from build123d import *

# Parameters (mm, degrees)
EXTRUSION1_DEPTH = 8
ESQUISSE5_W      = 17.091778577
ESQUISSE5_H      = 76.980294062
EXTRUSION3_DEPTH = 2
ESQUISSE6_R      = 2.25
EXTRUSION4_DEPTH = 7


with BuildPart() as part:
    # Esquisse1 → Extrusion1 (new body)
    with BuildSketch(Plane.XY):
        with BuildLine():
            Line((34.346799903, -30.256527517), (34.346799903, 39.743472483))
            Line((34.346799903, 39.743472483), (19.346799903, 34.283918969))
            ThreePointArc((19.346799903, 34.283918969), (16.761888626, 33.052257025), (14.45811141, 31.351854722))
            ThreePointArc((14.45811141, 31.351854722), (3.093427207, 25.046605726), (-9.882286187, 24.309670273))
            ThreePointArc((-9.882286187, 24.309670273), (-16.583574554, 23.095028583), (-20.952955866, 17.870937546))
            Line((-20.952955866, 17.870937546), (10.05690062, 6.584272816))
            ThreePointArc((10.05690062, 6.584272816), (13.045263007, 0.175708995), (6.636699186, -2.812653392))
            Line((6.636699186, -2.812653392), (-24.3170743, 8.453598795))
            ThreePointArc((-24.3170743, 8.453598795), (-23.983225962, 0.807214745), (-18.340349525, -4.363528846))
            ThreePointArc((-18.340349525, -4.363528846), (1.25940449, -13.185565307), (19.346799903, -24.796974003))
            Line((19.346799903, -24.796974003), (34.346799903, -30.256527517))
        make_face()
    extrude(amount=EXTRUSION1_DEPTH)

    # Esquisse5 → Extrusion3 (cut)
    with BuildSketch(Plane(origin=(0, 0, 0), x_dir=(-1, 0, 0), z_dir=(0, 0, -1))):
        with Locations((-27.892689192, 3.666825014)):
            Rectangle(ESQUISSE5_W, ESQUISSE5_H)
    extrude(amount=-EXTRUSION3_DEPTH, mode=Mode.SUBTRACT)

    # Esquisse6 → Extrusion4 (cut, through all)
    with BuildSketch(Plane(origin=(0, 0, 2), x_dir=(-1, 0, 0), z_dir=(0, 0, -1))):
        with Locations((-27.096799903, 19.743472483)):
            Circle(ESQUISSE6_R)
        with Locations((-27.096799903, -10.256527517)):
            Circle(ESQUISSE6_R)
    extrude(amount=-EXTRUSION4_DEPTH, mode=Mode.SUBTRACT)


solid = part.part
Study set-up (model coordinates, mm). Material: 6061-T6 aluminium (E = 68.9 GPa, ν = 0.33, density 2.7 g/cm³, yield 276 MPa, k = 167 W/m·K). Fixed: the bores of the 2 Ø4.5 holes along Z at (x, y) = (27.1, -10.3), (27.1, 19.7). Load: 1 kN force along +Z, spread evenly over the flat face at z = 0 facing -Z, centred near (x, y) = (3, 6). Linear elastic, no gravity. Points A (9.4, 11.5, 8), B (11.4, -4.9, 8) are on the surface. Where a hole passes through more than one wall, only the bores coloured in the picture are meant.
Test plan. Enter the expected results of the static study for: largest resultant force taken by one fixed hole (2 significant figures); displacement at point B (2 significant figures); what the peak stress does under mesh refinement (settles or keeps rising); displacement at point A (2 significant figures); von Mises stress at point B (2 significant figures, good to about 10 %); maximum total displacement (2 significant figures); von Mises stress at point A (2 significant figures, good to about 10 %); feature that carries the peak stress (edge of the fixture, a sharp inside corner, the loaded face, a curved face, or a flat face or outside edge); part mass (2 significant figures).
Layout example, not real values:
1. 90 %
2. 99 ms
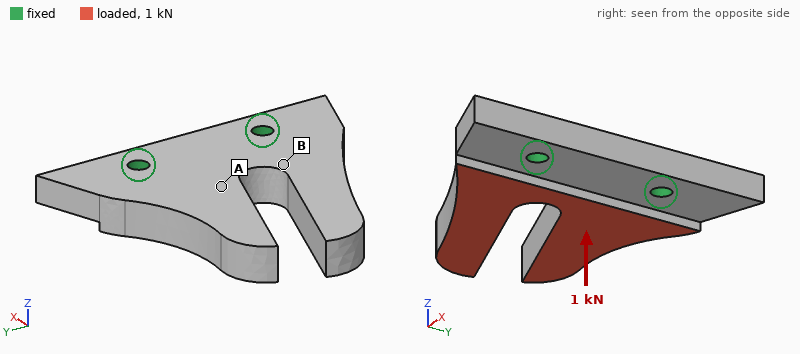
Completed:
1. 520 N
2. 0.049 mm
3. keeps rising
4. 0.050 mm
5. 43 MPa
6. 0.27 mm
7. 14 MPa
8. edge of the fixture
9. 42 g
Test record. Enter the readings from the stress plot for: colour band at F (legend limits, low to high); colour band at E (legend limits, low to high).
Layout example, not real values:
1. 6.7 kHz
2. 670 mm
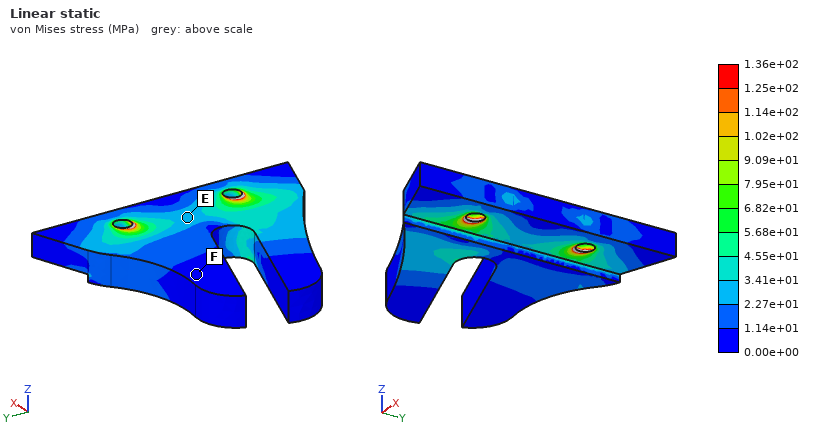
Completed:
1. 0.00e+00 to 1.14e+01 MPa
2. 2.27e+01 to 3.41e+01 MPa
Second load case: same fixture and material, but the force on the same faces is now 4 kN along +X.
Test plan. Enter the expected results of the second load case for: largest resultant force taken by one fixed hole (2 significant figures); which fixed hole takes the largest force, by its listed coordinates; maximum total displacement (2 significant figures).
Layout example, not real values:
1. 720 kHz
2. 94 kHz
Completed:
1. 2.2 kN
2. (27.1, 19.7)
3. 0.27 mm
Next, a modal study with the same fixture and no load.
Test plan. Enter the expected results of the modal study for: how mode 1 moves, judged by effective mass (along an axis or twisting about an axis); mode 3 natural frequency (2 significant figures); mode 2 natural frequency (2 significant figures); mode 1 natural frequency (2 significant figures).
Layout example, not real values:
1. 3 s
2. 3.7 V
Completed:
1. along Z
2. 5500 Hz
3. 3900 Hz
4. 2600 Hz
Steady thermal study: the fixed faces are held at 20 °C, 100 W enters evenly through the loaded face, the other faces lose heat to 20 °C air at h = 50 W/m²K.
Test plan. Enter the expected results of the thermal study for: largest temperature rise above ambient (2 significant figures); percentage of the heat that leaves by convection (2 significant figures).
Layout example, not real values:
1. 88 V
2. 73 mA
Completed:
1. 66 K
2. 6.6 %
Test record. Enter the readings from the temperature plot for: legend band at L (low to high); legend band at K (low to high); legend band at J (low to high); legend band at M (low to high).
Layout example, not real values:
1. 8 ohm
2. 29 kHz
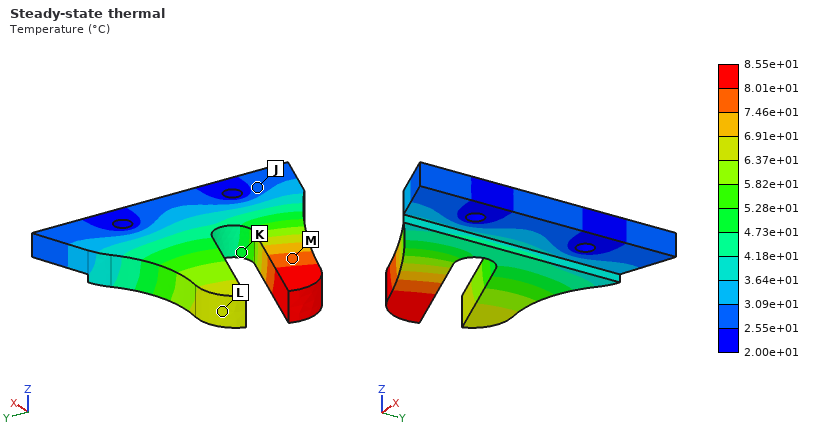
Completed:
1. 6.37e+01 to 6.91e+01 °C
2. 4.73e+01 to 5.28e+01 °C
3. 2.55e+01 to 3.09e+01 °C
4. 7.46e+01 to 8.01e+01 °C
